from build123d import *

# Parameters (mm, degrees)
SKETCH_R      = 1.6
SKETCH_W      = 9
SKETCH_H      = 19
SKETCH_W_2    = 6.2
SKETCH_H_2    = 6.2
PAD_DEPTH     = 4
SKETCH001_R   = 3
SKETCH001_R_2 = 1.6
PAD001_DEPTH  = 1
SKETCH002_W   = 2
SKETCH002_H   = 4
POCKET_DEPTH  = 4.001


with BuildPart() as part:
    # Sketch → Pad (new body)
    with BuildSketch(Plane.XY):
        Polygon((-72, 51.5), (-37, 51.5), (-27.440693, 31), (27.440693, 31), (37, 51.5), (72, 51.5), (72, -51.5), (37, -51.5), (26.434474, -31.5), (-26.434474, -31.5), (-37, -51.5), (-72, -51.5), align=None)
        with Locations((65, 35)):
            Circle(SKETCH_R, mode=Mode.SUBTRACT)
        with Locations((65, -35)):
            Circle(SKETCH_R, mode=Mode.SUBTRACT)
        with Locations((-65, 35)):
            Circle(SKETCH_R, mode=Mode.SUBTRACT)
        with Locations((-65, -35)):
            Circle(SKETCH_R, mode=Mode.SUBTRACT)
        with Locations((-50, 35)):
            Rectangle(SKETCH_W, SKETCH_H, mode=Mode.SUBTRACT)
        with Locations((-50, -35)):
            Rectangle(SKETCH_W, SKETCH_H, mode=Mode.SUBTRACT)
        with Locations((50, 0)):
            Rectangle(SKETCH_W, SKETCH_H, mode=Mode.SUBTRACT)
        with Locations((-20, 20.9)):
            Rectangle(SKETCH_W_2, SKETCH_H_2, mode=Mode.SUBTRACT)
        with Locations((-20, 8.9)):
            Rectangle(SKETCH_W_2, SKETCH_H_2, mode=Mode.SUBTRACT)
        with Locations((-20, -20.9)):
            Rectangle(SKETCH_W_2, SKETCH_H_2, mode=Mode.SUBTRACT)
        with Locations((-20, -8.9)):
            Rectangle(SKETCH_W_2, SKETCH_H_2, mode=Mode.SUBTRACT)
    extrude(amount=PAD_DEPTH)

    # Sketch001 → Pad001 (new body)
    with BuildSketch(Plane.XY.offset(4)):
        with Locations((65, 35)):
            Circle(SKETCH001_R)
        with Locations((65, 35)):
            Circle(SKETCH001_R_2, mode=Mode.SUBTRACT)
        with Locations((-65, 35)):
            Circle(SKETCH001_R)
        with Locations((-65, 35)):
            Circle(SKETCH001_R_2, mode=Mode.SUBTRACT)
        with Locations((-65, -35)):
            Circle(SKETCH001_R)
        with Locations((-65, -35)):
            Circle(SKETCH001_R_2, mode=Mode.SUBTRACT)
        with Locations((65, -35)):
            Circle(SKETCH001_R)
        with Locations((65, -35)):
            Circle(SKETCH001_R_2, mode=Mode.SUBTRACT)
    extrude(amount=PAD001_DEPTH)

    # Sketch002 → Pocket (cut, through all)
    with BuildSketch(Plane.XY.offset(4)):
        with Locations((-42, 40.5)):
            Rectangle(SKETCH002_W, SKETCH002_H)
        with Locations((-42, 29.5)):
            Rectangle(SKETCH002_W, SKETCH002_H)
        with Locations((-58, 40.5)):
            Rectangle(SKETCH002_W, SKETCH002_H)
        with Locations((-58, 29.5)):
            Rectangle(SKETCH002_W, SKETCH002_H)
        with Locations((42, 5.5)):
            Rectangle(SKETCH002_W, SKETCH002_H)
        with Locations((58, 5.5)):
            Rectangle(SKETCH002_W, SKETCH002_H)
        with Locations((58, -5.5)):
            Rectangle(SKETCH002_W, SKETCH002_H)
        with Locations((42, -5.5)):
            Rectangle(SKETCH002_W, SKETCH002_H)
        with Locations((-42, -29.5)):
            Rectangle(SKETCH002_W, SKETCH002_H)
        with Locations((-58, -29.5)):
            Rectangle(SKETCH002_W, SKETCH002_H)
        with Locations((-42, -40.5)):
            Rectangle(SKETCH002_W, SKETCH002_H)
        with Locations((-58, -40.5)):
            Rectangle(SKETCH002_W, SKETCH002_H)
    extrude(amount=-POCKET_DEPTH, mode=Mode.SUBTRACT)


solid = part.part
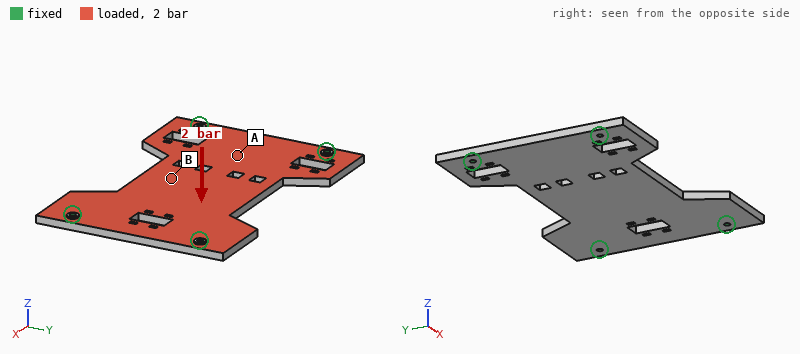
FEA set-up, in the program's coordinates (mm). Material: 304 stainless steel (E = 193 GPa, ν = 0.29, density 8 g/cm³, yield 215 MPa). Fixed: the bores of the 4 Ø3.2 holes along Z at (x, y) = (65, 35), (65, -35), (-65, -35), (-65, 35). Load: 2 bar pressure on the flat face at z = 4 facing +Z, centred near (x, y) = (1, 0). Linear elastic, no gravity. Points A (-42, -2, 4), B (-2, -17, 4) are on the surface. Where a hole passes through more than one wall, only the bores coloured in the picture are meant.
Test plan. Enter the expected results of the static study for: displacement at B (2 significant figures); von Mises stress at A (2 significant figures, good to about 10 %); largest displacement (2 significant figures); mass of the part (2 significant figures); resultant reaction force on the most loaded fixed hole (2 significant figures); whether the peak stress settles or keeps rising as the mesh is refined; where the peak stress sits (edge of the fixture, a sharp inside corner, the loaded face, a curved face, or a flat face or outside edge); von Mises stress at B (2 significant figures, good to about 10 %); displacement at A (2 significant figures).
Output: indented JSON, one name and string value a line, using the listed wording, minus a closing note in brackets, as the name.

{
  "displacement at B": "0.21 mm",
  "von Mises stress at A": "25 MPa",
  "largest displacement": "0.21 mm",
  "mass of the part": "370 g",
  "resultant reaction force on the most loaded fixed hole": "600 N",
  "whether the peak stress settles or keeps rising as the mesh is refined": "keeps rising",
  "where the peak stress sits": "edge of the fixture",
  "von Mises stress at B": "54 MPa",
  "displacement at A": "0.11 mm"
}
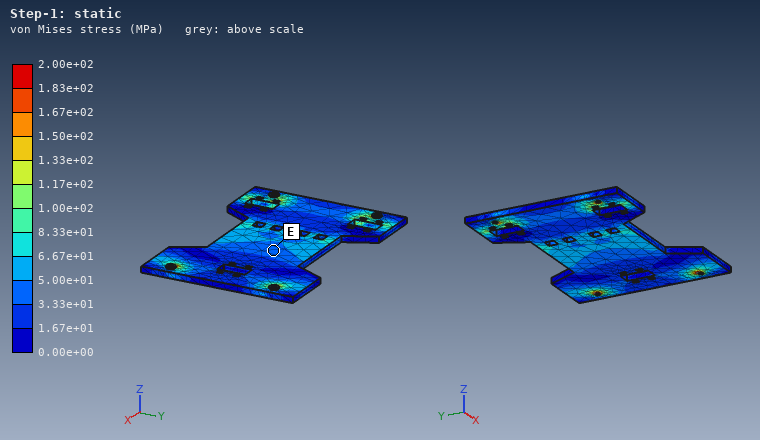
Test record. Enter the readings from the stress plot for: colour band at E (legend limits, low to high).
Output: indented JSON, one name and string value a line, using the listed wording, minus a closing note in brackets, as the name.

{
  "colour band at E": "3.33e+01 to 5.00e+01 MPa"
}
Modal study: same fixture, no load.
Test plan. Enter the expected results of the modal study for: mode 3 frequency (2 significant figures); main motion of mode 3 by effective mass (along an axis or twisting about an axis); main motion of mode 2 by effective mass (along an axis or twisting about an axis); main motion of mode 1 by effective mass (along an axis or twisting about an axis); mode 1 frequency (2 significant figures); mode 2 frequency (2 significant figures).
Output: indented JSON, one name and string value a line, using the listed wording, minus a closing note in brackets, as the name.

{
  "mode 3 frequency": "2500 Hz",
  "main motion of mode 3 by effective mass": "twisting about Y",
  "main motion of mode 2 by effective mass": "twisting about X",
  "main motion of mode 1 by effective mass": "along Z",
  "mode 1 frequency": "1000 Hz",
  "mode 2 frequency": "2000 Hz"
}
